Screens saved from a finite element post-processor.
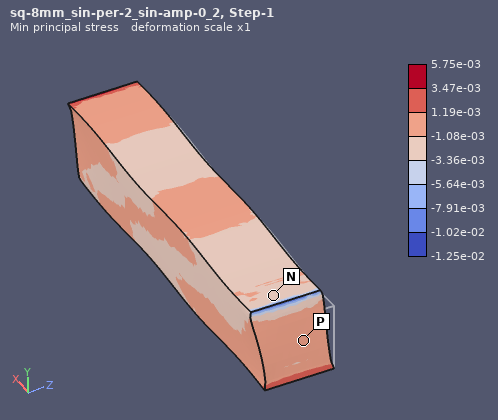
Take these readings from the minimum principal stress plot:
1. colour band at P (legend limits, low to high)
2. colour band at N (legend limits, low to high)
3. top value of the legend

-1.08e-03 to 1.19e-03
-3.36e-03 to -1.08e-03
5.75e-03
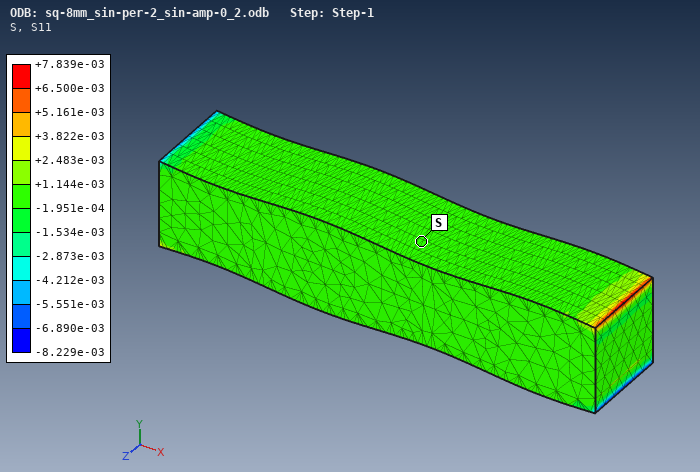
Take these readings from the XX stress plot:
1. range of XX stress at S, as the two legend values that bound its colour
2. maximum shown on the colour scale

-1.951e-04 to +1.144e-03
+7.839e-03
